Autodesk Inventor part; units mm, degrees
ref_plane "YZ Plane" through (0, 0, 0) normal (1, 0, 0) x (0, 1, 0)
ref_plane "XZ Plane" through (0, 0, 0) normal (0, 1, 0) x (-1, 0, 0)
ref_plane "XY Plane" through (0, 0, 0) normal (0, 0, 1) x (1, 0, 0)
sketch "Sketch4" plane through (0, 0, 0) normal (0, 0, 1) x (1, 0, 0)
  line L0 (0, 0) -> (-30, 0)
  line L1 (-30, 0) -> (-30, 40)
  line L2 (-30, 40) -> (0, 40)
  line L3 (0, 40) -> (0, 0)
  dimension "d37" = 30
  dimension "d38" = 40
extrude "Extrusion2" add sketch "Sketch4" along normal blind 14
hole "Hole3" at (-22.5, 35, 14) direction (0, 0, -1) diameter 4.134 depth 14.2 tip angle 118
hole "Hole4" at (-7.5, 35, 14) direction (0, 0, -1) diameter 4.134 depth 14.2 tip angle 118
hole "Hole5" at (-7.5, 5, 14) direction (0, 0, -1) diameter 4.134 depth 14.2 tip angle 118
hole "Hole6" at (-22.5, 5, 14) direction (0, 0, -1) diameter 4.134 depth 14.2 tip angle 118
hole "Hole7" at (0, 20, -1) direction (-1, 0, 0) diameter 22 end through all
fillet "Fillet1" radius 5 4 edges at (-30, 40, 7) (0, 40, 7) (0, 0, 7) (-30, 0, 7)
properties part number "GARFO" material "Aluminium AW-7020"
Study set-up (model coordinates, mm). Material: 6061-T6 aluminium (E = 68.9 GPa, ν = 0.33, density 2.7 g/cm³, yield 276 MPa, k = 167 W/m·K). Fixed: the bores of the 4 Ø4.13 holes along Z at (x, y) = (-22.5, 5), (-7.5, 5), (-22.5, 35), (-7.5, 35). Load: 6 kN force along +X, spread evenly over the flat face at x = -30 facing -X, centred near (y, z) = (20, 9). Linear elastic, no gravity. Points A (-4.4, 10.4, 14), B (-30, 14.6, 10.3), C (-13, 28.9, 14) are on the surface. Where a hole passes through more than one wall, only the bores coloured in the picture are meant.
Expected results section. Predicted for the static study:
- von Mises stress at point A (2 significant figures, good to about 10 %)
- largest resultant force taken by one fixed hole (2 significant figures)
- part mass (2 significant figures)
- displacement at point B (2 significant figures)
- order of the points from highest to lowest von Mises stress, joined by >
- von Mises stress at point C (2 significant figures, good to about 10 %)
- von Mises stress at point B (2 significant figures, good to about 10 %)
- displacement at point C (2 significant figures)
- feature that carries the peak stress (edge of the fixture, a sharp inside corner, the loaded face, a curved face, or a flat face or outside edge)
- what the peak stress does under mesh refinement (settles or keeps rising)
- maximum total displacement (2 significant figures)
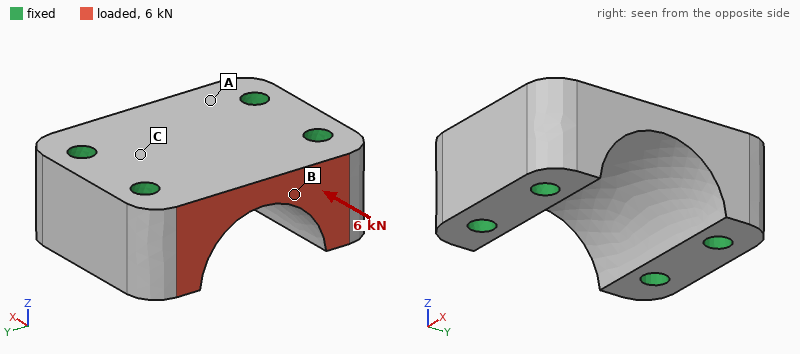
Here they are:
7.0 MPa
2.3 kN
29 g
6.3 µm
B > C > A
16 MPa
24 MPa
1.6 µm
edge of the fixture
keeps rising
8.2 µm
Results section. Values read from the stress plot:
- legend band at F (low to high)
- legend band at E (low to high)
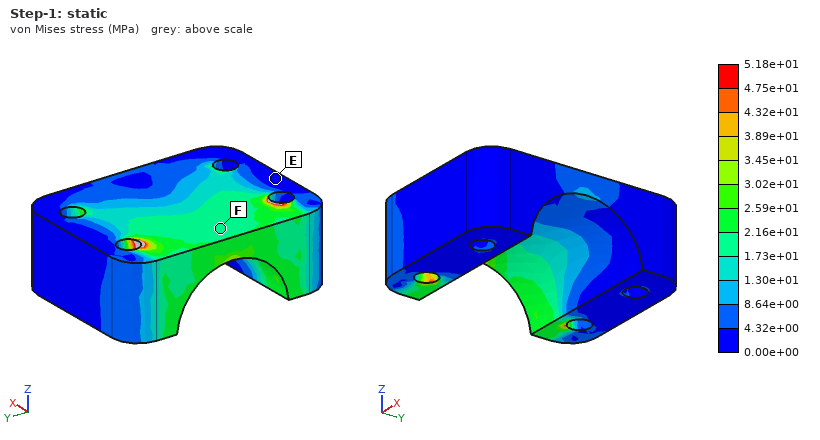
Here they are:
1.73e+01 to 2.16e+01 MPa
0.00e+00 to 4.32e+00 MPa
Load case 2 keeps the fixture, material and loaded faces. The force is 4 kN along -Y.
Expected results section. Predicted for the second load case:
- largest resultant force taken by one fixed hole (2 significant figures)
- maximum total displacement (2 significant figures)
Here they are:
2.1 kN
6.3 µm
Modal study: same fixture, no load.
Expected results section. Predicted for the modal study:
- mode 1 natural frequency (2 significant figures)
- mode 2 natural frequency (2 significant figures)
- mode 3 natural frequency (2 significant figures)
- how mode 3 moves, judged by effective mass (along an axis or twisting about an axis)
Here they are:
48 kHz
49 kHz
59 kHz
along X
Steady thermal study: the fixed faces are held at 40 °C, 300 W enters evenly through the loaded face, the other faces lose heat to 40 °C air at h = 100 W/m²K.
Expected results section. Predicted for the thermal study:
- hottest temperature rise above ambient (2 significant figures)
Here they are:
72 K
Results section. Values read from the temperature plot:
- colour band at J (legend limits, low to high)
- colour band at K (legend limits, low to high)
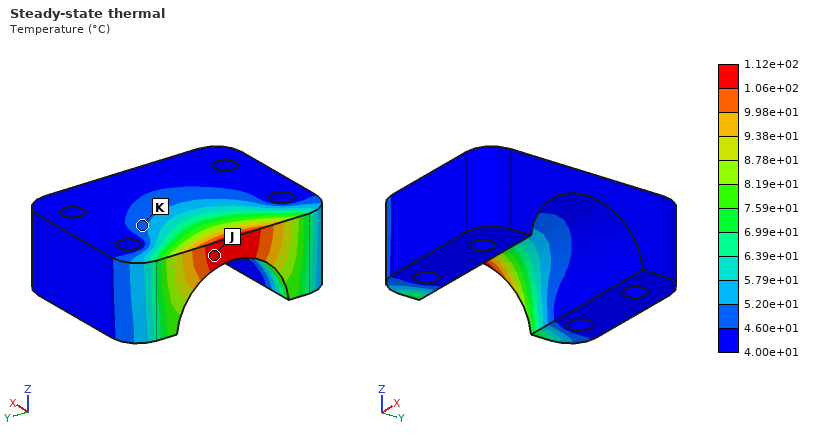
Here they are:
1.06e+02 to 1.12e+02 °C
4.60e+01 to 5.20e+01 °C
